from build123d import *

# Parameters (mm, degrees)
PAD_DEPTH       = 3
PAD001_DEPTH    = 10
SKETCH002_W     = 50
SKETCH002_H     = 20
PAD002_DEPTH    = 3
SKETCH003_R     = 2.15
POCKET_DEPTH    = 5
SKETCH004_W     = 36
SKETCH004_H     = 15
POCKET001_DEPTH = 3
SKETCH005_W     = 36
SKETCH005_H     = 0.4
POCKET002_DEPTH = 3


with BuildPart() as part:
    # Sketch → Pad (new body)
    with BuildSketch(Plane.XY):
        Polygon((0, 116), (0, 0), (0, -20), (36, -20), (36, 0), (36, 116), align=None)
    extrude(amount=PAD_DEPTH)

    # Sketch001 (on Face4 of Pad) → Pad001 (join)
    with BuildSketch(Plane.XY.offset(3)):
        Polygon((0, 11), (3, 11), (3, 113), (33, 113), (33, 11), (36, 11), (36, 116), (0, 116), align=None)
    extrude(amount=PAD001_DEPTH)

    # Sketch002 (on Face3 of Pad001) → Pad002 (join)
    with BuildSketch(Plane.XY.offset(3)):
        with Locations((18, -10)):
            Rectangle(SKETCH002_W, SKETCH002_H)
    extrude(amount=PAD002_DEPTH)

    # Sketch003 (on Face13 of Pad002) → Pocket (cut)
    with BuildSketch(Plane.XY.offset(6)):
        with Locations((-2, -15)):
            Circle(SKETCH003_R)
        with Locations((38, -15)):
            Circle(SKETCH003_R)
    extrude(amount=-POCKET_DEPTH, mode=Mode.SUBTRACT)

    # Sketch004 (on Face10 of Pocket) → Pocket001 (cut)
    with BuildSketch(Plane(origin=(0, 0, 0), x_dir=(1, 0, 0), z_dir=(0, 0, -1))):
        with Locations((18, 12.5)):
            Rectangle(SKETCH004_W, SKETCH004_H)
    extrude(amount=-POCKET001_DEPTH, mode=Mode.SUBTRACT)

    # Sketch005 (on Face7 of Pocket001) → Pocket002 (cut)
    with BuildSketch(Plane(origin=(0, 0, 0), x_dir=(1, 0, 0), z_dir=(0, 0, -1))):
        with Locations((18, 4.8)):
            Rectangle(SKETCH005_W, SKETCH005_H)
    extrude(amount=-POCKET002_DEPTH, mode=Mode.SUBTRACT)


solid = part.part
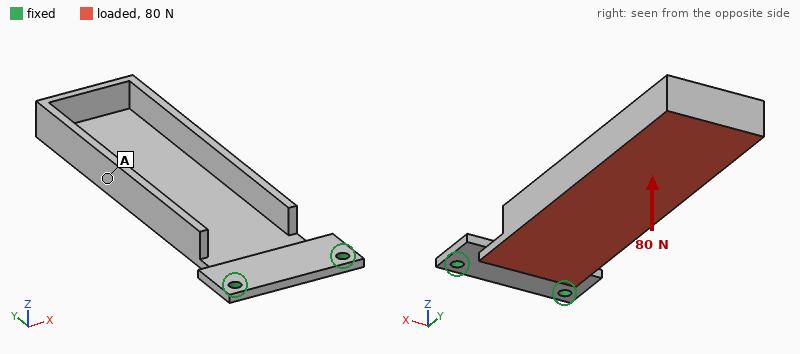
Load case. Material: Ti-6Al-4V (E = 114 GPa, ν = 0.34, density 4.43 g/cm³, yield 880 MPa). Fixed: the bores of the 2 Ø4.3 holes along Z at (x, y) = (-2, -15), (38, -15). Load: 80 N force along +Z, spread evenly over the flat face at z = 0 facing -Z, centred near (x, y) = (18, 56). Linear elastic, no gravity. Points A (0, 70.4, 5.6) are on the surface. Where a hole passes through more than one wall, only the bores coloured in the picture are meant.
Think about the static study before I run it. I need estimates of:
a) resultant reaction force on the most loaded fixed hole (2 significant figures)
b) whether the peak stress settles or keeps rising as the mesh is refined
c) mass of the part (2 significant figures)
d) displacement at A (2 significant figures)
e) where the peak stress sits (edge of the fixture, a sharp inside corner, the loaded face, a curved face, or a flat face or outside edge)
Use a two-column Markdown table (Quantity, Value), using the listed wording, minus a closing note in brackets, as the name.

| Quantity | Value |
|---|---|
| resultant reaction force on the most loaded fixed hole | 43 N |
| whether the peak stress settles or keeps rising as the mesh is refined | keeps rising |
| mass of the part | 100 g |
| displacement at A | 0.96 mm |
| where the peak stress sits | edge of the fixture |
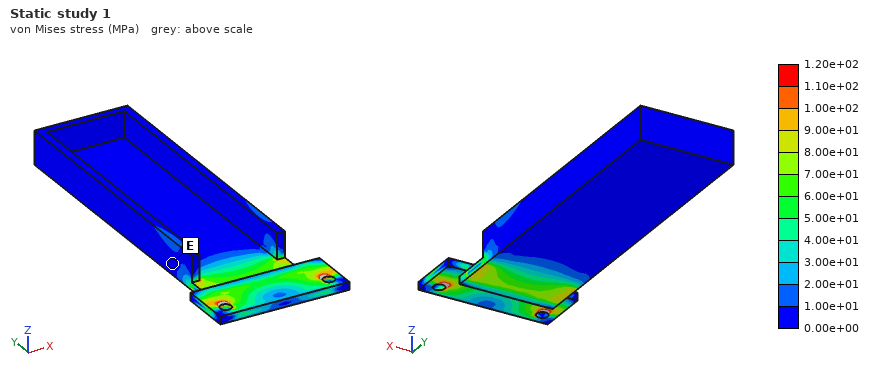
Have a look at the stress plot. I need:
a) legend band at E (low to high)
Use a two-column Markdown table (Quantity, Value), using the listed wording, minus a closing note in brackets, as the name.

| Quantity | Value |
|---|---|
| legend band at E | 0.00e+00 to 1.00e+01 MPa |
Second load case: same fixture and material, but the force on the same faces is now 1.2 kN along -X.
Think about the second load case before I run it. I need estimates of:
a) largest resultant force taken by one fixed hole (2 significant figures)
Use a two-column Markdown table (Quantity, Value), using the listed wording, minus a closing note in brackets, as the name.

| Quantity | Value |
|---|---|
| largest resultant force taken by one fixed hole | 2.2 kN |
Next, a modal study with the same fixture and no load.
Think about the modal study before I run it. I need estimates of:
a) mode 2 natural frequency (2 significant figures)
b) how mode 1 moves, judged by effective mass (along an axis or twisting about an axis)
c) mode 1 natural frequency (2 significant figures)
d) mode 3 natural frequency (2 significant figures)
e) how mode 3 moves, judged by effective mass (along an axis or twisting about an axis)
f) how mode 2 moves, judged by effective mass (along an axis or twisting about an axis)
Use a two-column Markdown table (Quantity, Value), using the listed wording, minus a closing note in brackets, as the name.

| Quantity | Value |
|---|---|
| mode 2 natural frequency | 770 Hz |
| how mode 1 moves, judged by effective mass | along Z |
| mode 1 natural frequency | 140 Hz |
| mode 3 natural frequency | 1200 Hz |
| how mode 3 moves, judged by effective mass | along X |
| how mode 2 moves, judged by effective mass | along X |
